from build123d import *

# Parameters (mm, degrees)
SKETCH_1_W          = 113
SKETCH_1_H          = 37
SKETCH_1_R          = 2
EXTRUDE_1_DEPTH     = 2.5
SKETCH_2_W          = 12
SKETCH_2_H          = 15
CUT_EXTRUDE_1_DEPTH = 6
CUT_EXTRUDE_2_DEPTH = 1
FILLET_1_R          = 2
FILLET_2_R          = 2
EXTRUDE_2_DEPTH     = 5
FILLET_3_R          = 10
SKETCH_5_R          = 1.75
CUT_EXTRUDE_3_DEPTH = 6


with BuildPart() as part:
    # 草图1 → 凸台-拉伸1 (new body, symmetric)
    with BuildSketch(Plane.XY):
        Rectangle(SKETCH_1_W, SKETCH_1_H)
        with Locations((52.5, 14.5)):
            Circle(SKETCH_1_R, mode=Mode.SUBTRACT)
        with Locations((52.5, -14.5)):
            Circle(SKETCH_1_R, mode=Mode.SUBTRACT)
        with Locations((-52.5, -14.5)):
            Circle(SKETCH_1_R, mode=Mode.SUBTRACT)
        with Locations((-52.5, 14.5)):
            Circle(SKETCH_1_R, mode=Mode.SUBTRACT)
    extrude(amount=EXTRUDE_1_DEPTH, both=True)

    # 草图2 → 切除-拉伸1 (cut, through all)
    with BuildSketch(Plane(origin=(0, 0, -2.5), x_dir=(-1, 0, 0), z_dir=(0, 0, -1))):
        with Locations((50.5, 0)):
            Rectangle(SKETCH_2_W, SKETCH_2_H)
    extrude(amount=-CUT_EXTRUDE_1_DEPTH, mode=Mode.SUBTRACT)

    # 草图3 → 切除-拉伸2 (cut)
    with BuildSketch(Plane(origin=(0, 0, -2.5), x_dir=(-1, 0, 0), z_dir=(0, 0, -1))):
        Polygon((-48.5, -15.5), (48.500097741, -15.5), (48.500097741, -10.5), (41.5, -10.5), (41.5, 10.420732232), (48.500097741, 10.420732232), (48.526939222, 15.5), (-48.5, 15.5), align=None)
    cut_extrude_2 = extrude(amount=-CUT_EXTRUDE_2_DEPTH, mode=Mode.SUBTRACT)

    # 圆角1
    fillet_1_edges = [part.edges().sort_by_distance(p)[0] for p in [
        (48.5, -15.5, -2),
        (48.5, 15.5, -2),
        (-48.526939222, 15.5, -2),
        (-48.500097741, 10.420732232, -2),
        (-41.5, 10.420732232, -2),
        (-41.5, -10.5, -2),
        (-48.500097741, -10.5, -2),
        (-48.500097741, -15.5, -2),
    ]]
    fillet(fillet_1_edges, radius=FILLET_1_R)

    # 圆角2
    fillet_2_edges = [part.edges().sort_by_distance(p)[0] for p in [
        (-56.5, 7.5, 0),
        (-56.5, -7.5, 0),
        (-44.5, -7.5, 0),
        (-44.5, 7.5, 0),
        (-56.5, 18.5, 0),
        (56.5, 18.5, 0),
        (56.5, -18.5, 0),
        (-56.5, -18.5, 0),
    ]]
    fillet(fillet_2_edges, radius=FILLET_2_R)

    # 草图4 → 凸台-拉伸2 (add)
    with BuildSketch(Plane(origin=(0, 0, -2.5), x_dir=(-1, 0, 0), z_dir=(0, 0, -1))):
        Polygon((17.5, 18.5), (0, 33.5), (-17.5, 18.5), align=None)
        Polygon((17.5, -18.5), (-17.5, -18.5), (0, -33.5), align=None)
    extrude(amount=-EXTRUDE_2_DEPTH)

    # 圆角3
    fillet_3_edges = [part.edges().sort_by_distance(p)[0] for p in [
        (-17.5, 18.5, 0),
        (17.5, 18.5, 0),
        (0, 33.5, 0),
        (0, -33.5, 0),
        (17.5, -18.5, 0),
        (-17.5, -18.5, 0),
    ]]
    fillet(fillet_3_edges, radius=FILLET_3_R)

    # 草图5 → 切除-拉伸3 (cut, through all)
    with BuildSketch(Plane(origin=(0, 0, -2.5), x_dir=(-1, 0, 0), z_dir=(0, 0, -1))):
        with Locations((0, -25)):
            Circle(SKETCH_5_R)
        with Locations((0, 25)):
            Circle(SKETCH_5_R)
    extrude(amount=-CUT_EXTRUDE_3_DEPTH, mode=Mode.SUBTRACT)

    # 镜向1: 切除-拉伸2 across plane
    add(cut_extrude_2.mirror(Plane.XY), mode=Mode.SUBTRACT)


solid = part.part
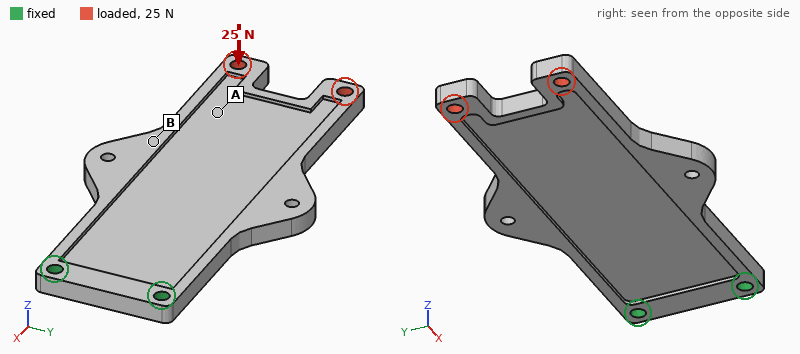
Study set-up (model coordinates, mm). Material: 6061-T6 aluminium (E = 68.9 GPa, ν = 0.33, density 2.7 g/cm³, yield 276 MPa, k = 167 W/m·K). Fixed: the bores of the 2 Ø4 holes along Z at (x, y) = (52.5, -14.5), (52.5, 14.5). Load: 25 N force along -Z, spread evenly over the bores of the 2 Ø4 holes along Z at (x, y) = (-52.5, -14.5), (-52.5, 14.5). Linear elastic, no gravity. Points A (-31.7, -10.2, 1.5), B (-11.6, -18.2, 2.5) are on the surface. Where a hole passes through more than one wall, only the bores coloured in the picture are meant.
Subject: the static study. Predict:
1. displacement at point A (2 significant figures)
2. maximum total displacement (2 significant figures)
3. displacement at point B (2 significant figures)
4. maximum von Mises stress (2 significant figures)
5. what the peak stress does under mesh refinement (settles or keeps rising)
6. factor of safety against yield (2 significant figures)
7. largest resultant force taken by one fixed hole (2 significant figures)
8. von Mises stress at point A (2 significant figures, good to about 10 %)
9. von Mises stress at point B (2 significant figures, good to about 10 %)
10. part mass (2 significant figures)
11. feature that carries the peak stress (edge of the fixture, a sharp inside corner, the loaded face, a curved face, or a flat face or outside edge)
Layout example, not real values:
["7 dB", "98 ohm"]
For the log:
["0.63 mm", "0.93 mm", "0.40 mm", "57 MPa", "settles", "4.8", "13 N", "6.1 MPa", "12 MPa", "44 g", "a curved face"]
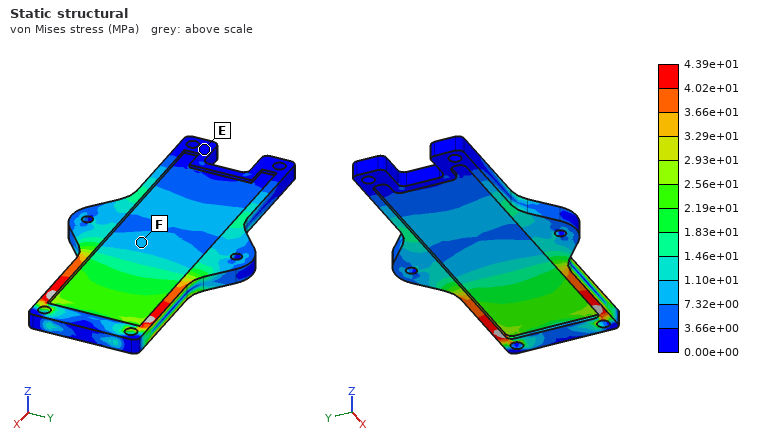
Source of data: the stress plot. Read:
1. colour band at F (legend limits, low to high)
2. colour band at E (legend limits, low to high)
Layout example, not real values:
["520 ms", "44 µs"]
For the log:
["7.32e+00 to 1.10e+01 MPa", "0.00e+00 to 3.66e+00 MPa"]
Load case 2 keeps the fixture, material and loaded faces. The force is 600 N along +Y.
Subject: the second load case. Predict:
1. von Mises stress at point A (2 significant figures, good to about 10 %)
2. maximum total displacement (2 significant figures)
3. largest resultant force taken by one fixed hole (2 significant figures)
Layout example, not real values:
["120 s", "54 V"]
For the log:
["8.9 MPa", "0.23 mm", "2.1 kN"]
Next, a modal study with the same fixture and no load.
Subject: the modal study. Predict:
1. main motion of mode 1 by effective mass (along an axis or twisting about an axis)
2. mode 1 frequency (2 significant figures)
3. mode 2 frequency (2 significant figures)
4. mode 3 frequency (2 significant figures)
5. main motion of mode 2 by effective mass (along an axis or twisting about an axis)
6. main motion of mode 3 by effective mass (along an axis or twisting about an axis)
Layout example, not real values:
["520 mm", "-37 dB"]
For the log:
["along Z", "270 Hz", "1100 Hz", "1600 Hz", "twisting about X", "along Z"]
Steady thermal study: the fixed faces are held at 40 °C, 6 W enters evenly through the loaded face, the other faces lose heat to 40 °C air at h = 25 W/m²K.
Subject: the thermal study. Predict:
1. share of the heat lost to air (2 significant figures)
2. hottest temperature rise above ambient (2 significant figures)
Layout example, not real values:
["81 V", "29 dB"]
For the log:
["42 %", "22 K"]
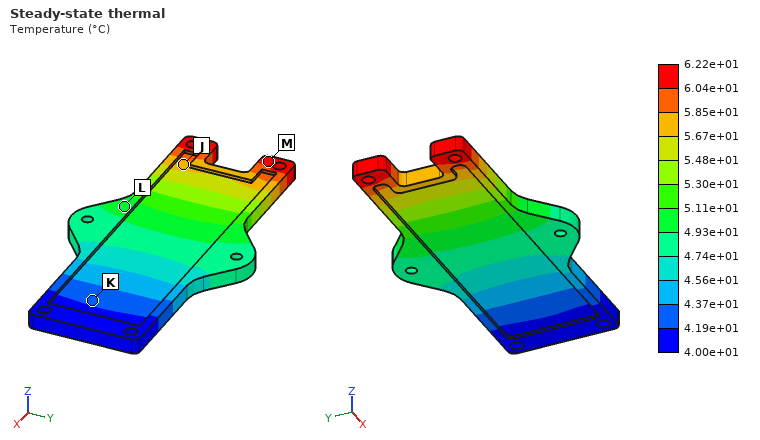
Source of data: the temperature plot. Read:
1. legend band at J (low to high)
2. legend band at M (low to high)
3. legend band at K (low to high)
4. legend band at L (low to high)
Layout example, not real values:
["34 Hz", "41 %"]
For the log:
["5.67e+01 to 5.85e+01 °C", "6.04e+01 to 6.22e+01 °C", "4.19e+01 to 4.37e+01 °C", "4.93e+01 to 5.11e+01 °C"]
